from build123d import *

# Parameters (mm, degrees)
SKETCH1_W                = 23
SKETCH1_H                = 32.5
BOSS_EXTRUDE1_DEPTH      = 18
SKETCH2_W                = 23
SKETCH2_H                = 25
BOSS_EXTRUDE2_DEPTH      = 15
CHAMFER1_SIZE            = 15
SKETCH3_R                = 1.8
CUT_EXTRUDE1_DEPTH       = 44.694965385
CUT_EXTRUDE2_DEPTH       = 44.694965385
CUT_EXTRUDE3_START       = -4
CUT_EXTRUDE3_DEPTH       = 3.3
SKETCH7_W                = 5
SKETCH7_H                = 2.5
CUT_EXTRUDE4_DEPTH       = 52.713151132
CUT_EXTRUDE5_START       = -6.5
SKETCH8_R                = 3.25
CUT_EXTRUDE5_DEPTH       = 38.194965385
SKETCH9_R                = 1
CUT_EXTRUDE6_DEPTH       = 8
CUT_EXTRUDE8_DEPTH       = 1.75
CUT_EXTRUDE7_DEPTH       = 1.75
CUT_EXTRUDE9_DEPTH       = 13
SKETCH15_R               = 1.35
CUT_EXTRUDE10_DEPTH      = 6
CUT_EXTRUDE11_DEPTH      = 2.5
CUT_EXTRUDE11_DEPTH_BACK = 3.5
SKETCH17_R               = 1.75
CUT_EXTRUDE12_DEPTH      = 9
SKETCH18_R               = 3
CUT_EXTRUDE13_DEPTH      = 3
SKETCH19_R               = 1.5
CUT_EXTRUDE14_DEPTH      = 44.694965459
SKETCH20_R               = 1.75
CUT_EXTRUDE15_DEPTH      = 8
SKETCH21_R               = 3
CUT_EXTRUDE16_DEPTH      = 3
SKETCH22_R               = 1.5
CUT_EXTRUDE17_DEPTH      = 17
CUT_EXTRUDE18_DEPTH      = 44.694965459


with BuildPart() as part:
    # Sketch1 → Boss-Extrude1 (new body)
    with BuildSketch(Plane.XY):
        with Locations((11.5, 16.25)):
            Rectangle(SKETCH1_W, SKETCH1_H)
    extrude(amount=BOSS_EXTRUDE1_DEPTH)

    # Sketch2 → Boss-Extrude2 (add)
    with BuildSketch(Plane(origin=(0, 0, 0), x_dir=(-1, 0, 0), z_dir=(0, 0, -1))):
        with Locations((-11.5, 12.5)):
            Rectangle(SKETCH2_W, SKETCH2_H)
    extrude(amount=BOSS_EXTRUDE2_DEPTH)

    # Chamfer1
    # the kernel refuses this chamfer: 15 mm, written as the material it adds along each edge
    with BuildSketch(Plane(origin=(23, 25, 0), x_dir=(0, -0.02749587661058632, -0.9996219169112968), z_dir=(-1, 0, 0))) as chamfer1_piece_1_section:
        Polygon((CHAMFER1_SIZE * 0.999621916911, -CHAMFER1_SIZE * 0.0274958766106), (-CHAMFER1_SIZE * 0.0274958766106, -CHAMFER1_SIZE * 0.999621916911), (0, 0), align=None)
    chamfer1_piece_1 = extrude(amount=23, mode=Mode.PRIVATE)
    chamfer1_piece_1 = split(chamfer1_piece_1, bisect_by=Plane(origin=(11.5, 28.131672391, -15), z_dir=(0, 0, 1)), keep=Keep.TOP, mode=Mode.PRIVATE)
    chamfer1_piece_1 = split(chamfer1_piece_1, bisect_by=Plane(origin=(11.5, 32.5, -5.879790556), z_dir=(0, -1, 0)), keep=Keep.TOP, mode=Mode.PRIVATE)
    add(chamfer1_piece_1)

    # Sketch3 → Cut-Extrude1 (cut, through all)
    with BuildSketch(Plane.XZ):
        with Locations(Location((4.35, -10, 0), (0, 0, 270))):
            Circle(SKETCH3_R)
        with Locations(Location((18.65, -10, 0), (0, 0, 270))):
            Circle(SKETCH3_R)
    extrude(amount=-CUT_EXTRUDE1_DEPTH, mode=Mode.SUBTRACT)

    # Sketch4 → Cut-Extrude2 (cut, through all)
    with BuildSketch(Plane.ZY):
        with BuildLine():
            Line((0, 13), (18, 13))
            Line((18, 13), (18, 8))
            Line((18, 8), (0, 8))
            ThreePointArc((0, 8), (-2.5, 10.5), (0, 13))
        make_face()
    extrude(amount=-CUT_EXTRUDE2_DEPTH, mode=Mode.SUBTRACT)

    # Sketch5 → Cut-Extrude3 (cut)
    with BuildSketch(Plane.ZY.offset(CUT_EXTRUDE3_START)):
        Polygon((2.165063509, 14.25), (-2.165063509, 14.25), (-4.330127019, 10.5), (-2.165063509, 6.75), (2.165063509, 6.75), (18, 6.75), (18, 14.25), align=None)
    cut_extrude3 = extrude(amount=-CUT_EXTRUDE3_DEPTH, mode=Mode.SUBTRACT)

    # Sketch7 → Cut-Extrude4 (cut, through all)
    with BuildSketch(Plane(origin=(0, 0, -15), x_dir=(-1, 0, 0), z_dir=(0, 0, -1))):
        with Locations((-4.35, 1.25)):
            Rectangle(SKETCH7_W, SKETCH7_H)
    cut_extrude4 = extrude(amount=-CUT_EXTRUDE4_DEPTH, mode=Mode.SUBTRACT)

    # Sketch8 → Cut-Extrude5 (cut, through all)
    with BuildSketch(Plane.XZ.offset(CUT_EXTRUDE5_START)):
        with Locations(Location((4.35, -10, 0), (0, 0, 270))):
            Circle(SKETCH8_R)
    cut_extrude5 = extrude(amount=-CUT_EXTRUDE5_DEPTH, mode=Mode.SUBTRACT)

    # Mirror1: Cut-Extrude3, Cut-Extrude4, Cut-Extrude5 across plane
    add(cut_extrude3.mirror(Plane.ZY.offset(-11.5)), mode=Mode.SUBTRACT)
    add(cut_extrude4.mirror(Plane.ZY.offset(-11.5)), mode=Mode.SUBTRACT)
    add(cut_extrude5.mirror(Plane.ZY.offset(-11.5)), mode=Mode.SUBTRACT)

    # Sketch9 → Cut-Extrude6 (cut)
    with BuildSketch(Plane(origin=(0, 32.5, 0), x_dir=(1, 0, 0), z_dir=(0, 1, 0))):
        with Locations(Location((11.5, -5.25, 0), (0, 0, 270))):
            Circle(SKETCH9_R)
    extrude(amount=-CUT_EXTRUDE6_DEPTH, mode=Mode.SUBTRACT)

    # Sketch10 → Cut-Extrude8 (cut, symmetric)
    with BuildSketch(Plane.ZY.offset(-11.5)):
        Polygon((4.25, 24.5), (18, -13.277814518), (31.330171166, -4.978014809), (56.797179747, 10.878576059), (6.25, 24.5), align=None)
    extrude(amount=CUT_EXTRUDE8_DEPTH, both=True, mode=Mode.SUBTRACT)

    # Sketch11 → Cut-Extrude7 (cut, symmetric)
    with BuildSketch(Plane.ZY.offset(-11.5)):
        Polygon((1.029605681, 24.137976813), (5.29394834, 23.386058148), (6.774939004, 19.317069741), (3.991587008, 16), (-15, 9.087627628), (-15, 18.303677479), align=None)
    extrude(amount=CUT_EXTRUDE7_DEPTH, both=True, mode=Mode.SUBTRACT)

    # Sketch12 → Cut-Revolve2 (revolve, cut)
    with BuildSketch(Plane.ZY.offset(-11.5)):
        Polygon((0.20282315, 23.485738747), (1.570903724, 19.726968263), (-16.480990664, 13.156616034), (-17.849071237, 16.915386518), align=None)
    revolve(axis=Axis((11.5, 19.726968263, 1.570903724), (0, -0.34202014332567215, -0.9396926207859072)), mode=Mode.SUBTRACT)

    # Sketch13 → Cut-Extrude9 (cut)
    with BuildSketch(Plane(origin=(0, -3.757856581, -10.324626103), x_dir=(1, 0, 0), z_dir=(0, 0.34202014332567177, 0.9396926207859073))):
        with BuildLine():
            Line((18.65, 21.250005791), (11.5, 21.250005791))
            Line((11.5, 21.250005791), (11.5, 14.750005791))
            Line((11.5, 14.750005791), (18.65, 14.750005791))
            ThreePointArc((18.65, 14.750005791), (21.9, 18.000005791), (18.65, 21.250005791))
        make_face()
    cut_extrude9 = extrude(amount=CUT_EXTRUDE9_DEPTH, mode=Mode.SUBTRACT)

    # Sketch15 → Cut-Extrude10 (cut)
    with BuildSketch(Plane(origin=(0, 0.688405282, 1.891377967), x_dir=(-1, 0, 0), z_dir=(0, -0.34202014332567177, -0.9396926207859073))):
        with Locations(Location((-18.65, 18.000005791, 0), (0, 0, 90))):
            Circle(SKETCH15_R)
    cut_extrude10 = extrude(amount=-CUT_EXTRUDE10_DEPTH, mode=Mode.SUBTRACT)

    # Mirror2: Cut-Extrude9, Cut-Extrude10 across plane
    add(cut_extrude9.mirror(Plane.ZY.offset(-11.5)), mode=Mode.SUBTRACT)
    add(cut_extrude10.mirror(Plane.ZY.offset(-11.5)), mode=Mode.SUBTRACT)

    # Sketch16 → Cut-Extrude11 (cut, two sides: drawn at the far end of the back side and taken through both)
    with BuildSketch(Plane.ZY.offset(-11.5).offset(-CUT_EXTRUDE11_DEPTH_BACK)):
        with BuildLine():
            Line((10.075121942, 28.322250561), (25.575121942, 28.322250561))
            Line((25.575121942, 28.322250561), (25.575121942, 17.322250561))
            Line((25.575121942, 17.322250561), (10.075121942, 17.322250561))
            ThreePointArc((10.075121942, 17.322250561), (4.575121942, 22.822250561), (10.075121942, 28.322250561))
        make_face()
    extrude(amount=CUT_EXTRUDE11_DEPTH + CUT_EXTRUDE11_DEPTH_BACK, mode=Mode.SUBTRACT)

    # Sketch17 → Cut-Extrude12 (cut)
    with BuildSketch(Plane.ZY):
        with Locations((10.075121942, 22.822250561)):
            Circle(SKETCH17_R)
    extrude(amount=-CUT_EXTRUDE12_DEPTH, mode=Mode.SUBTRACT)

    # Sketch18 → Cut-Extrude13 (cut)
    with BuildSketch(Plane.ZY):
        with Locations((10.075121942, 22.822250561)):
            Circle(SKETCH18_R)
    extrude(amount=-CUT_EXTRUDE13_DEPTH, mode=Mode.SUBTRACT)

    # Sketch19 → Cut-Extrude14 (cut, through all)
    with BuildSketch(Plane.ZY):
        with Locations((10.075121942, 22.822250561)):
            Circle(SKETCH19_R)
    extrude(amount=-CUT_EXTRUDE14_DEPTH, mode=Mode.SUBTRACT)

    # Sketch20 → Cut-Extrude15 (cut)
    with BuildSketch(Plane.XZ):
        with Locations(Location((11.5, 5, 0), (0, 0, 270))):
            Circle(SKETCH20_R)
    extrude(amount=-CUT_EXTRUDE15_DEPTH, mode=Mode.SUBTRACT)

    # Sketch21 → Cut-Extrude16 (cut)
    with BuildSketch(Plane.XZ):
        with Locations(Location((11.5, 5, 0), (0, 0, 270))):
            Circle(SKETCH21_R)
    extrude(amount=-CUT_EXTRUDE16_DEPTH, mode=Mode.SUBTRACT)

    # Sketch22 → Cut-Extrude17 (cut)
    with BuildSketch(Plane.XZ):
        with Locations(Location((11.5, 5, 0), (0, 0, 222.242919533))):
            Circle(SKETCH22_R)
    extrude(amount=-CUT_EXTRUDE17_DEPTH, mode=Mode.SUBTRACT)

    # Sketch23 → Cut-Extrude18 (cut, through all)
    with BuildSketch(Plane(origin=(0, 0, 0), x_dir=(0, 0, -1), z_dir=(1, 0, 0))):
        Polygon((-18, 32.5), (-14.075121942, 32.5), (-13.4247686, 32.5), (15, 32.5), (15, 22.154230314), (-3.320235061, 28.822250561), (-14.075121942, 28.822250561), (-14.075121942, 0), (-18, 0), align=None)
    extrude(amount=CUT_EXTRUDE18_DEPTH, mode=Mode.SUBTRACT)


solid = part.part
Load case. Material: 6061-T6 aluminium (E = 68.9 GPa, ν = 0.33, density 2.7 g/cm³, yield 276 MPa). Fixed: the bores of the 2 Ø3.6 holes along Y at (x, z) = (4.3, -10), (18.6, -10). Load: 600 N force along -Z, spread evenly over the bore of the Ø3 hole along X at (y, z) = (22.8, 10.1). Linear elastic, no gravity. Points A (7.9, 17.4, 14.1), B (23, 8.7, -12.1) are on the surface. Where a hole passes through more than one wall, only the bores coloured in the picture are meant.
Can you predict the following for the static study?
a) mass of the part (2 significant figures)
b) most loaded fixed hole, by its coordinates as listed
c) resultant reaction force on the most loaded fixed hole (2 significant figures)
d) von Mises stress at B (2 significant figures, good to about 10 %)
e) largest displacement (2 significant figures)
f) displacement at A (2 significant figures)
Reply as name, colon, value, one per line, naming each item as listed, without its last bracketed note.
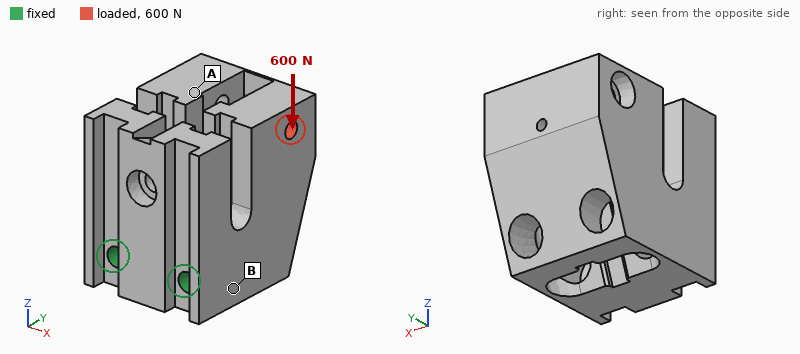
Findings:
mass of the part: 30 g
most loaded fixed hole, by its coordinates as listed: (18.6, -10)
resultant reaction force on the most loaded fixed hole: 570 N
von Mises stress at B: 35 MPa
largest displacement: 99 µm
displacement at A: 67 µm
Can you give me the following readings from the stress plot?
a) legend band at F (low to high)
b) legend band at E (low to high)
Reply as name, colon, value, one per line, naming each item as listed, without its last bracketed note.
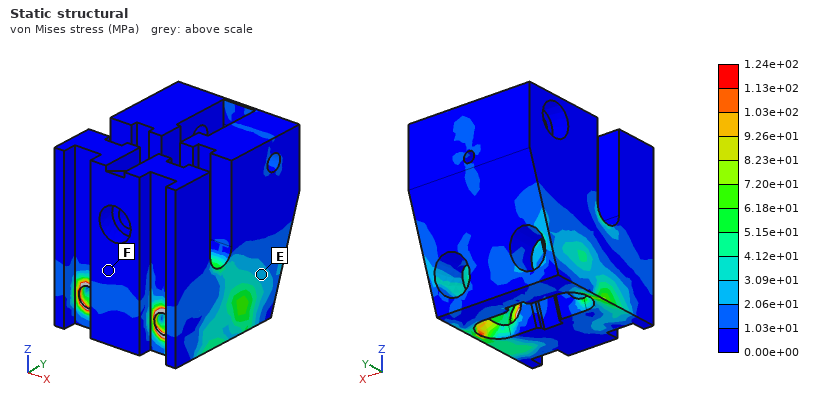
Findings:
legend band at F: 0.00e+00 to 1.03e+01 MPa
legend band at E: 2.06e+01 to 3.09e+01 MPa
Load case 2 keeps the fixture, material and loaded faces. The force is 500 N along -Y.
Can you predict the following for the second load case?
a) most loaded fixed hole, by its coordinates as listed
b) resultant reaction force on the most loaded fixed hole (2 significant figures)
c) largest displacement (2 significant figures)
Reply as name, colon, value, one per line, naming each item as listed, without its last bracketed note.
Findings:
most loaded fixed hole, by its coordinates as listed: (18.6, -10)
resultant reaction force on the most loaded fixed hole: 480 N
largest displacement: 0.10 mm
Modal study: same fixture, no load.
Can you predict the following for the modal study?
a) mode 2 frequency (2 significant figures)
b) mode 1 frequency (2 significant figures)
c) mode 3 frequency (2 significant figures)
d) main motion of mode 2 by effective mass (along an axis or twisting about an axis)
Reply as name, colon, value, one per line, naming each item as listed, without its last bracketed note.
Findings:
mode 2 frequency: 8000 Hz
mode 1 frequency: 3600 Hz
mode 3 frequency: 9500 Hz
main motion of mode 2 by effective mass: along X
